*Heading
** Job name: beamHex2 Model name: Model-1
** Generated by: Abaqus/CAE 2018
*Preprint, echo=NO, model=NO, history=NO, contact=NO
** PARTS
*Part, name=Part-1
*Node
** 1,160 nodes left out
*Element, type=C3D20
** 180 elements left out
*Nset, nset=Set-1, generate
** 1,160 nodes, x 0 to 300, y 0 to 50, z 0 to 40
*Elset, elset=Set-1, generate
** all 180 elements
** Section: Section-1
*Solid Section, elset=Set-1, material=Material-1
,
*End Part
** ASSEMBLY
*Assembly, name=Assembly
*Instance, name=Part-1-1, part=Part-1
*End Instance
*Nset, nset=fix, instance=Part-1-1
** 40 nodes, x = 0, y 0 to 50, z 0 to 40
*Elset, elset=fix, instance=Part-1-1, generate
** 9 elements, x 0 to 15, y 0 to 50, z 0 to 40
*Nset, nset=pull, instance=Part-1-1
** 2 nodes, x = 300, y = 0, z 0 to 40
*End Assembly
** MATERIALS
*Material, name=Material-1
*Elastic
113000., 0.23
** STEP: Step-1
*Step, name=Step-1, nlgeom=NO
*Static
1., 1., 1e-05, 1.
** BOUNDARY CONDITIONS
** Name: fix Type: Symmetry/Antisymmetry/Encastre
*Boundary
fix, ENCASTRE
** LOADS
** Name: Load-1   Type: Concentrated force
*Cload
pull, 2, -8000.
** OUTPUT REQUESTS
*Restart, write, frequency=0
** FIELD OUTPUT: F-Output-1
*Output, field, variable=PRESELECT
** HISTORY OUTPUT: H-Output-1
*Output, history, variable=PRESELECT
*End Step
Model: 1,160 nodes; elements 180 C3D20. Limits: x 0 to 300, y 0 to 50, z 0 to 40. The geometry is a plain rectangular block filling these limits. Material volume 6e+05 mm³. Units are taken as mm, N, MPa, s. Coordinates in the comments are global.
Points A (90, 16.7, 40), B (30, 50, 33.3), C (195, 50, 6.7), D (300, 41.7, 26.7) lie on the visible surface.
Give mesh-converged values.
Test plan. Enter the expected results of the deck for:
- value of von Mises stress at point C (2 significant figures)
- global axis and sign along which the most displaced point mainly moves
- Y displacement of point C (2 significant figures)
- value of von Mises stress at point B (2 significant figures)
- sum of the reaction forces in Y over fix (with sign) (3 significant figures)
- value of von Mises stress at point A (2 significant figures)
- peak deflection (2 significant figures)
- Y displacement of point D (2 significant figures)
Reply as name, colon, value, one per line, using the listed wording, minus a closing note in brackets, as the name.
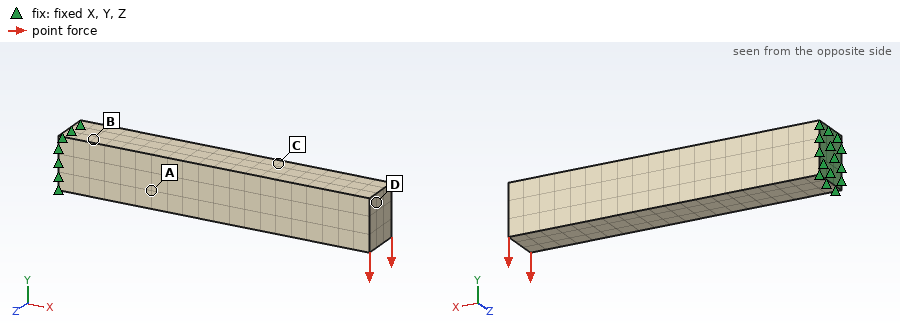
value of von Mises stress at point C: 100 MPa
global axis and sign along which the most displaced point mainly moves: -Y
Y displacement of point C: -1.5 mm
value of von Mises stress at point B: 260 MPa
sum of the reaction forces in Y over fix (with sign): 16000 N
value of von Mises stress at point A: 70 MPa
peak deflection: 3.3 mm
Y displacement of point D: -3.1 mm
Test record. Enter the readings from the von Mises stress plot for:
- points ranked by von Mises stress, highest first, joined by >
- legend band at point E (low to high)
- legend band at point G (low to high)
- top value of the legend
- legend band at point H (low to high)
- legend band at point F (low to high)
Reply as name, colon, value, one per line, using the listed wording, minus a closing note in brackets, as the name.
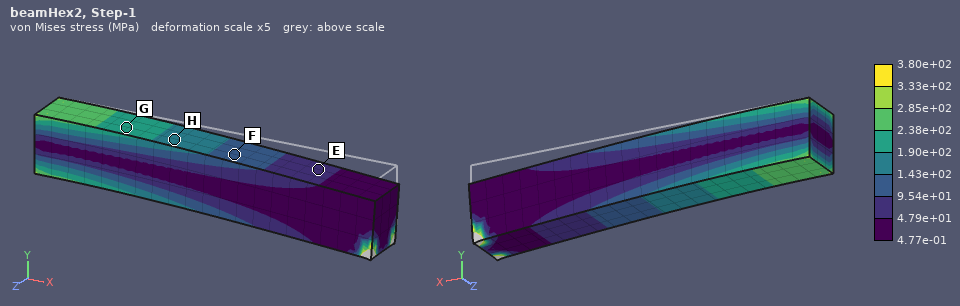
points ranked by von Mises stress, highest first, joined by >: G > H > F > E
legend band at point E: 4.79e+01 to 9.54e+01 MPa
legend band at point G: 1.90e+02 to 2.38e+02 MPa
top value of the legend: 3.80e+02 MPa
legend band at point H: 1.43e+02 to 1.90e+02 MPa
legend band at point F: 9.54e+01 to 1.43e+02 MPa
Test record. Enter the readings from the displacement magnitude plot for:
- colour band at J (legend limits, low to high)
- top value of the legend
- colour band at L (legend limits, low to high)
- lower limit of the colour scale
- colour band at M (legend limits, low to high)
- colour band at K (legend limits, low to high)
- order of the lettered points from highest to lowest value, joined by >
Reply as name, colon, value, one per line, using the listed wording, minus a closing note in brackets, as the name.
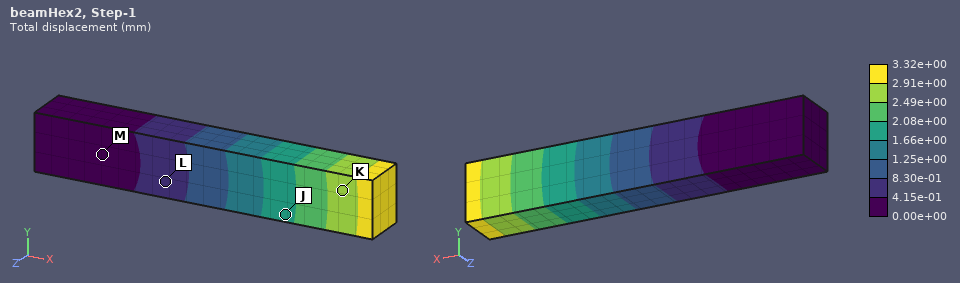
colour band at J: 1.66e+00 to 2.08e+00 mm
top value of the legend: 3.32e+00 mm
colour band at L: 4.15e-01 to 8.30e-01 mm
lower limit of the colour scale: 0.00e+00 mm
colour band at M: 0.00e+00 to 4.15e-01 mm
colour band at K: 2.49e+00 to 2.91e+00 mm
order of the lettered points from highest to lowest value, joined by >: K > J > L > M
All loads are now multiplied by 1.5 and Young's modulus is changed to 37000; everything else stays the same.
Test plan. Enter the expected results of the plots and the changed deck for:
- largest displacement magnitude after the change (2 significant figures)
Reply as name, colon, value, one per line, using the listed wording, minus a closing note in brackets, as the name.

largest displacement magnitude after the change: 15 mm
